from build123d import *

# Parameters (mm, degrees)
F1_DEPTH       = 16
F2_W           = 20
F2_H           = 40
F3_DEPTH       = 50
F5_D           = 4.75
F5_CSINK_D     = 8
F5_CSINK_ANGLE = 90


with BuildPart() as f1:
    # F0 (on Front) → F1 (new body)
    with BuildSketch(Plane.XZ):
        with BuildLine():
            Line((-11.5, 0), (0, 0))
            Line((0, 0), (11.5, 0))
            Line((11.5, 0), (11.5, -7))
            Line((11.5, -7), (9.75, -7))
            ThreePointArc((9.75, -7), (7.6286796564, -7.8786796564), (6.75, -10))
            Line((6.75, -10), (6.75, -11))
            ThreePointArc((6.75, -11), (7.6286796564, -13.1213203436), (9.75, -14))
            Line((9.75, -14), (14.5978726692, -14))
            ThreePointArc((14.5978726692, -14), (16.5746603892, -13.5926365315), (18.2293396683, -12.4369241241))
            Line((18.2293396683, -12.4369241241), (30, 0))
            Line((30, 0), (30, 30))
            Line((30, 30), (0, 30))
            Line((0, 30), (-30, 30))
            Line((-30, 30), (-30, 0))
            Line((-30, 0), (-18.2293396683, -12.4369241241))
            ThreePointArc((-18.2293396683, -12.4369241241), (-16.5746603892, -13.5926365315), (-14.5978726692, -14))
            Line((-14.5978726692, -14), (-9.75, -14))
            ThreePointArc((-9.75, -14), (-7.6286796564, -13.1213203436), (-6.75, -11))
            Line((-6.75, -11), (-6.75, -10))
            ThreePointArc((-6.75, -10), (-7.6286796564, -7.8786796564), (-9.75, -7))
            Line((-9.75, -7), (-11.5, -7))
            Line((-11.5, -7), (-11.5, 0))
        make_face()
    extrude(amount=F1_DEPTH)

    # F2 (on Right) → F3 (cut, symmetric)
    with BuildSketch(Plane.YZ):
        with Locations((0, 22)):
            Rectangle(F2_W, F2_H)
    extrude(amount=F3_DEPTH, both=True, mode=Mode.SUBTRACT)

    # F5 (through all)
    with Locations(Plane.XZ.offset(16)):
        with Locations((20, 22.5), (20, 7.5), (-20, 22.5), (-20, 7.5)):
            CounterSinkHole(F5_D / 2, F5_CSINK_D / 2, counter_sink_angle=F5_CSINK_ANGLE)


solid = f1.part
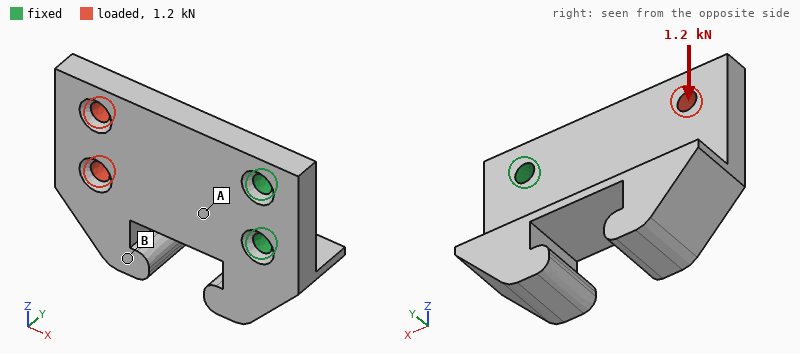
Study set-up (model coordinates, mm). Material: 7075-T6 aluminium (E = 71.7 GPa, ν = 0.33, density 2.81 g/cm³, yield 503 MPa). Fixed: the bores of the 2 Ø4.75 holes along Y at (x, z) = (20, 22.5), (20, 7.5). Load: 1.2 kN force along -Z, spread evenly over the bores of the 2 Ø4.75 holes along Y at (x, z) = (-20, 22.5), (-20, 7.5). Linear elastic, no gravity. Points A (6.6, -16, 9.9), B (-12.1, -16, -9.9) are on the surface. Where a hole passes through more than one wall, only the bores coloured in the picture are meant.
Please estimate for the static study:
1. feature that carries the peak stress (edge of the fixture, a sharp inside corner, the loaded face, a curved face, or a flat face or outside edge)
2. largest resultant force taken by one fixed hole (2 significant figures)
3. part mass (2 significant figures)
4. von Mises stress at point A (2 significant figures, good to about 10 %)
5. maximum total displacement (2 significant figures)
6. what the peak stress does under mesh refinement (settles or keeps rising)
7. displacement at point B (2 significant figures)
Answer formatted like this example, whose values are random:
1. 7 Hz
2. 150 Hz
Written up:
1. edge of the fixture
2. 2.7 kN
3. 50 g
4. 19 MPa
5. 73 µm
6. keeps rising
7. 50 µm
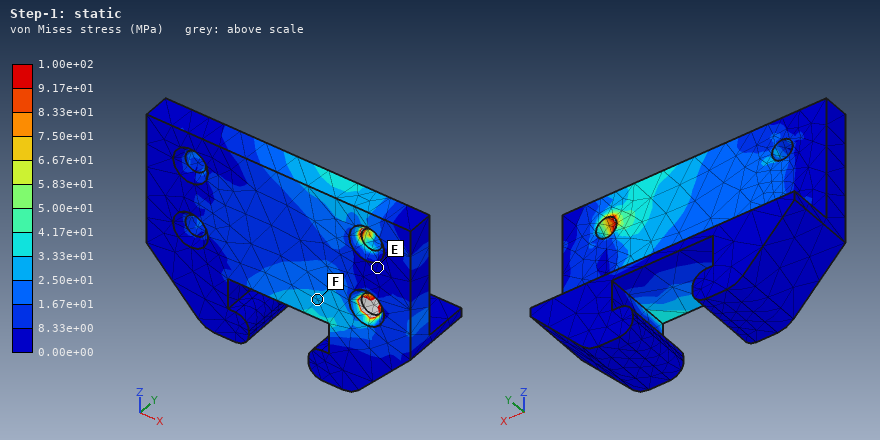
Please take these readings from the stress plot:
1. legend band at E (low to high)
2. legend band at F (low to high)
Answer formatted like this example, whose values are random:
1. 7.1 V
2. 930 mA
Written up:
1. 0.00e+00 to 8.33e+00 MPa
2. 2.50e+01 to 3.33e+01 MPa
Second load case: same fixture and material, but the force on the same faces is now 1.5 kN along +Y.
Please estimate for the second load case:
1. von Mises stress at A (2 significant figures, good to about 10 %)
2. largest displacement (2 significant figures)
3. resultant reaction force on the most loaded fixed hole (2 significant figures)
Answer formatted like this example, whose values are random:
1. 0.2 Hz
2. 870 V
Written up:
1. 110 MPa
2. 0.76 mm
3. 760 N
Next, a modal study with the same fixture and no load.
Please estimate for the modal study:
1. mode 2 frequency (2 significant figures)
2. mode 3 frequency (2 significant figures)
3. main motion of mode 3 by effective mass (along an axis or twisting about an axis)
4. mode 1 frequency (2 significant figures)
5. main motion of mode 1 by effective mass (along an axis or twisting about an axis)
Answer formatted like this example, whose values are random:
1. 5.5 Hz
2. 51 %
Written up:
1. 3400 Hz
2. 5400 Hz
3. along Z
4. 1800 Hz
5. along Y
